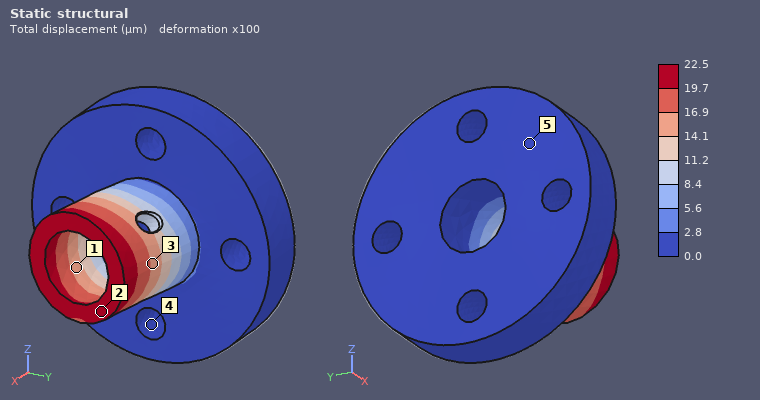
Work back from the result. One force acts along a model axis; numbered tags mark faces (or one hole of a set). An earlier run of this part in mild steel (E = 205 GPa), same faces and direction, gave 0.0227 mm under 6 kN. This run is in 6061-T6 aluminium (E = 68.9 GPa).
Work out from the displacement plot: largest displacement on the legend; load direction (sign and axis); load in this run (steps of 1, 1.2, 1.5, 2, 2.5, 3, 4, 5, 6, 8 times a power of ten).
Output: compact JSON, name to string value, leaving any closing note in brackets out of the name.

{"largest displacement on the legend": "22.5 µm", "load direction": "-Y", "load in this run": "2 kN"}
